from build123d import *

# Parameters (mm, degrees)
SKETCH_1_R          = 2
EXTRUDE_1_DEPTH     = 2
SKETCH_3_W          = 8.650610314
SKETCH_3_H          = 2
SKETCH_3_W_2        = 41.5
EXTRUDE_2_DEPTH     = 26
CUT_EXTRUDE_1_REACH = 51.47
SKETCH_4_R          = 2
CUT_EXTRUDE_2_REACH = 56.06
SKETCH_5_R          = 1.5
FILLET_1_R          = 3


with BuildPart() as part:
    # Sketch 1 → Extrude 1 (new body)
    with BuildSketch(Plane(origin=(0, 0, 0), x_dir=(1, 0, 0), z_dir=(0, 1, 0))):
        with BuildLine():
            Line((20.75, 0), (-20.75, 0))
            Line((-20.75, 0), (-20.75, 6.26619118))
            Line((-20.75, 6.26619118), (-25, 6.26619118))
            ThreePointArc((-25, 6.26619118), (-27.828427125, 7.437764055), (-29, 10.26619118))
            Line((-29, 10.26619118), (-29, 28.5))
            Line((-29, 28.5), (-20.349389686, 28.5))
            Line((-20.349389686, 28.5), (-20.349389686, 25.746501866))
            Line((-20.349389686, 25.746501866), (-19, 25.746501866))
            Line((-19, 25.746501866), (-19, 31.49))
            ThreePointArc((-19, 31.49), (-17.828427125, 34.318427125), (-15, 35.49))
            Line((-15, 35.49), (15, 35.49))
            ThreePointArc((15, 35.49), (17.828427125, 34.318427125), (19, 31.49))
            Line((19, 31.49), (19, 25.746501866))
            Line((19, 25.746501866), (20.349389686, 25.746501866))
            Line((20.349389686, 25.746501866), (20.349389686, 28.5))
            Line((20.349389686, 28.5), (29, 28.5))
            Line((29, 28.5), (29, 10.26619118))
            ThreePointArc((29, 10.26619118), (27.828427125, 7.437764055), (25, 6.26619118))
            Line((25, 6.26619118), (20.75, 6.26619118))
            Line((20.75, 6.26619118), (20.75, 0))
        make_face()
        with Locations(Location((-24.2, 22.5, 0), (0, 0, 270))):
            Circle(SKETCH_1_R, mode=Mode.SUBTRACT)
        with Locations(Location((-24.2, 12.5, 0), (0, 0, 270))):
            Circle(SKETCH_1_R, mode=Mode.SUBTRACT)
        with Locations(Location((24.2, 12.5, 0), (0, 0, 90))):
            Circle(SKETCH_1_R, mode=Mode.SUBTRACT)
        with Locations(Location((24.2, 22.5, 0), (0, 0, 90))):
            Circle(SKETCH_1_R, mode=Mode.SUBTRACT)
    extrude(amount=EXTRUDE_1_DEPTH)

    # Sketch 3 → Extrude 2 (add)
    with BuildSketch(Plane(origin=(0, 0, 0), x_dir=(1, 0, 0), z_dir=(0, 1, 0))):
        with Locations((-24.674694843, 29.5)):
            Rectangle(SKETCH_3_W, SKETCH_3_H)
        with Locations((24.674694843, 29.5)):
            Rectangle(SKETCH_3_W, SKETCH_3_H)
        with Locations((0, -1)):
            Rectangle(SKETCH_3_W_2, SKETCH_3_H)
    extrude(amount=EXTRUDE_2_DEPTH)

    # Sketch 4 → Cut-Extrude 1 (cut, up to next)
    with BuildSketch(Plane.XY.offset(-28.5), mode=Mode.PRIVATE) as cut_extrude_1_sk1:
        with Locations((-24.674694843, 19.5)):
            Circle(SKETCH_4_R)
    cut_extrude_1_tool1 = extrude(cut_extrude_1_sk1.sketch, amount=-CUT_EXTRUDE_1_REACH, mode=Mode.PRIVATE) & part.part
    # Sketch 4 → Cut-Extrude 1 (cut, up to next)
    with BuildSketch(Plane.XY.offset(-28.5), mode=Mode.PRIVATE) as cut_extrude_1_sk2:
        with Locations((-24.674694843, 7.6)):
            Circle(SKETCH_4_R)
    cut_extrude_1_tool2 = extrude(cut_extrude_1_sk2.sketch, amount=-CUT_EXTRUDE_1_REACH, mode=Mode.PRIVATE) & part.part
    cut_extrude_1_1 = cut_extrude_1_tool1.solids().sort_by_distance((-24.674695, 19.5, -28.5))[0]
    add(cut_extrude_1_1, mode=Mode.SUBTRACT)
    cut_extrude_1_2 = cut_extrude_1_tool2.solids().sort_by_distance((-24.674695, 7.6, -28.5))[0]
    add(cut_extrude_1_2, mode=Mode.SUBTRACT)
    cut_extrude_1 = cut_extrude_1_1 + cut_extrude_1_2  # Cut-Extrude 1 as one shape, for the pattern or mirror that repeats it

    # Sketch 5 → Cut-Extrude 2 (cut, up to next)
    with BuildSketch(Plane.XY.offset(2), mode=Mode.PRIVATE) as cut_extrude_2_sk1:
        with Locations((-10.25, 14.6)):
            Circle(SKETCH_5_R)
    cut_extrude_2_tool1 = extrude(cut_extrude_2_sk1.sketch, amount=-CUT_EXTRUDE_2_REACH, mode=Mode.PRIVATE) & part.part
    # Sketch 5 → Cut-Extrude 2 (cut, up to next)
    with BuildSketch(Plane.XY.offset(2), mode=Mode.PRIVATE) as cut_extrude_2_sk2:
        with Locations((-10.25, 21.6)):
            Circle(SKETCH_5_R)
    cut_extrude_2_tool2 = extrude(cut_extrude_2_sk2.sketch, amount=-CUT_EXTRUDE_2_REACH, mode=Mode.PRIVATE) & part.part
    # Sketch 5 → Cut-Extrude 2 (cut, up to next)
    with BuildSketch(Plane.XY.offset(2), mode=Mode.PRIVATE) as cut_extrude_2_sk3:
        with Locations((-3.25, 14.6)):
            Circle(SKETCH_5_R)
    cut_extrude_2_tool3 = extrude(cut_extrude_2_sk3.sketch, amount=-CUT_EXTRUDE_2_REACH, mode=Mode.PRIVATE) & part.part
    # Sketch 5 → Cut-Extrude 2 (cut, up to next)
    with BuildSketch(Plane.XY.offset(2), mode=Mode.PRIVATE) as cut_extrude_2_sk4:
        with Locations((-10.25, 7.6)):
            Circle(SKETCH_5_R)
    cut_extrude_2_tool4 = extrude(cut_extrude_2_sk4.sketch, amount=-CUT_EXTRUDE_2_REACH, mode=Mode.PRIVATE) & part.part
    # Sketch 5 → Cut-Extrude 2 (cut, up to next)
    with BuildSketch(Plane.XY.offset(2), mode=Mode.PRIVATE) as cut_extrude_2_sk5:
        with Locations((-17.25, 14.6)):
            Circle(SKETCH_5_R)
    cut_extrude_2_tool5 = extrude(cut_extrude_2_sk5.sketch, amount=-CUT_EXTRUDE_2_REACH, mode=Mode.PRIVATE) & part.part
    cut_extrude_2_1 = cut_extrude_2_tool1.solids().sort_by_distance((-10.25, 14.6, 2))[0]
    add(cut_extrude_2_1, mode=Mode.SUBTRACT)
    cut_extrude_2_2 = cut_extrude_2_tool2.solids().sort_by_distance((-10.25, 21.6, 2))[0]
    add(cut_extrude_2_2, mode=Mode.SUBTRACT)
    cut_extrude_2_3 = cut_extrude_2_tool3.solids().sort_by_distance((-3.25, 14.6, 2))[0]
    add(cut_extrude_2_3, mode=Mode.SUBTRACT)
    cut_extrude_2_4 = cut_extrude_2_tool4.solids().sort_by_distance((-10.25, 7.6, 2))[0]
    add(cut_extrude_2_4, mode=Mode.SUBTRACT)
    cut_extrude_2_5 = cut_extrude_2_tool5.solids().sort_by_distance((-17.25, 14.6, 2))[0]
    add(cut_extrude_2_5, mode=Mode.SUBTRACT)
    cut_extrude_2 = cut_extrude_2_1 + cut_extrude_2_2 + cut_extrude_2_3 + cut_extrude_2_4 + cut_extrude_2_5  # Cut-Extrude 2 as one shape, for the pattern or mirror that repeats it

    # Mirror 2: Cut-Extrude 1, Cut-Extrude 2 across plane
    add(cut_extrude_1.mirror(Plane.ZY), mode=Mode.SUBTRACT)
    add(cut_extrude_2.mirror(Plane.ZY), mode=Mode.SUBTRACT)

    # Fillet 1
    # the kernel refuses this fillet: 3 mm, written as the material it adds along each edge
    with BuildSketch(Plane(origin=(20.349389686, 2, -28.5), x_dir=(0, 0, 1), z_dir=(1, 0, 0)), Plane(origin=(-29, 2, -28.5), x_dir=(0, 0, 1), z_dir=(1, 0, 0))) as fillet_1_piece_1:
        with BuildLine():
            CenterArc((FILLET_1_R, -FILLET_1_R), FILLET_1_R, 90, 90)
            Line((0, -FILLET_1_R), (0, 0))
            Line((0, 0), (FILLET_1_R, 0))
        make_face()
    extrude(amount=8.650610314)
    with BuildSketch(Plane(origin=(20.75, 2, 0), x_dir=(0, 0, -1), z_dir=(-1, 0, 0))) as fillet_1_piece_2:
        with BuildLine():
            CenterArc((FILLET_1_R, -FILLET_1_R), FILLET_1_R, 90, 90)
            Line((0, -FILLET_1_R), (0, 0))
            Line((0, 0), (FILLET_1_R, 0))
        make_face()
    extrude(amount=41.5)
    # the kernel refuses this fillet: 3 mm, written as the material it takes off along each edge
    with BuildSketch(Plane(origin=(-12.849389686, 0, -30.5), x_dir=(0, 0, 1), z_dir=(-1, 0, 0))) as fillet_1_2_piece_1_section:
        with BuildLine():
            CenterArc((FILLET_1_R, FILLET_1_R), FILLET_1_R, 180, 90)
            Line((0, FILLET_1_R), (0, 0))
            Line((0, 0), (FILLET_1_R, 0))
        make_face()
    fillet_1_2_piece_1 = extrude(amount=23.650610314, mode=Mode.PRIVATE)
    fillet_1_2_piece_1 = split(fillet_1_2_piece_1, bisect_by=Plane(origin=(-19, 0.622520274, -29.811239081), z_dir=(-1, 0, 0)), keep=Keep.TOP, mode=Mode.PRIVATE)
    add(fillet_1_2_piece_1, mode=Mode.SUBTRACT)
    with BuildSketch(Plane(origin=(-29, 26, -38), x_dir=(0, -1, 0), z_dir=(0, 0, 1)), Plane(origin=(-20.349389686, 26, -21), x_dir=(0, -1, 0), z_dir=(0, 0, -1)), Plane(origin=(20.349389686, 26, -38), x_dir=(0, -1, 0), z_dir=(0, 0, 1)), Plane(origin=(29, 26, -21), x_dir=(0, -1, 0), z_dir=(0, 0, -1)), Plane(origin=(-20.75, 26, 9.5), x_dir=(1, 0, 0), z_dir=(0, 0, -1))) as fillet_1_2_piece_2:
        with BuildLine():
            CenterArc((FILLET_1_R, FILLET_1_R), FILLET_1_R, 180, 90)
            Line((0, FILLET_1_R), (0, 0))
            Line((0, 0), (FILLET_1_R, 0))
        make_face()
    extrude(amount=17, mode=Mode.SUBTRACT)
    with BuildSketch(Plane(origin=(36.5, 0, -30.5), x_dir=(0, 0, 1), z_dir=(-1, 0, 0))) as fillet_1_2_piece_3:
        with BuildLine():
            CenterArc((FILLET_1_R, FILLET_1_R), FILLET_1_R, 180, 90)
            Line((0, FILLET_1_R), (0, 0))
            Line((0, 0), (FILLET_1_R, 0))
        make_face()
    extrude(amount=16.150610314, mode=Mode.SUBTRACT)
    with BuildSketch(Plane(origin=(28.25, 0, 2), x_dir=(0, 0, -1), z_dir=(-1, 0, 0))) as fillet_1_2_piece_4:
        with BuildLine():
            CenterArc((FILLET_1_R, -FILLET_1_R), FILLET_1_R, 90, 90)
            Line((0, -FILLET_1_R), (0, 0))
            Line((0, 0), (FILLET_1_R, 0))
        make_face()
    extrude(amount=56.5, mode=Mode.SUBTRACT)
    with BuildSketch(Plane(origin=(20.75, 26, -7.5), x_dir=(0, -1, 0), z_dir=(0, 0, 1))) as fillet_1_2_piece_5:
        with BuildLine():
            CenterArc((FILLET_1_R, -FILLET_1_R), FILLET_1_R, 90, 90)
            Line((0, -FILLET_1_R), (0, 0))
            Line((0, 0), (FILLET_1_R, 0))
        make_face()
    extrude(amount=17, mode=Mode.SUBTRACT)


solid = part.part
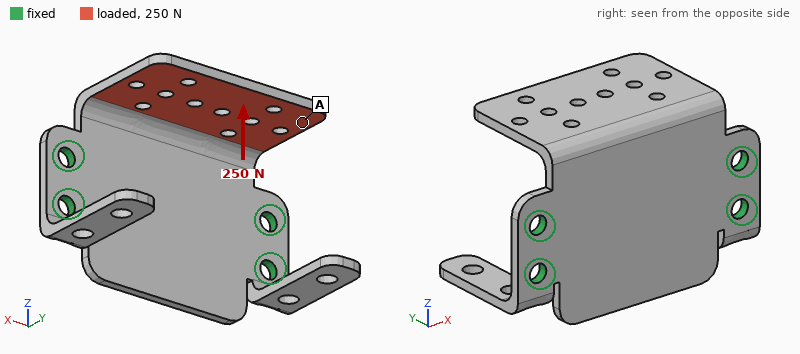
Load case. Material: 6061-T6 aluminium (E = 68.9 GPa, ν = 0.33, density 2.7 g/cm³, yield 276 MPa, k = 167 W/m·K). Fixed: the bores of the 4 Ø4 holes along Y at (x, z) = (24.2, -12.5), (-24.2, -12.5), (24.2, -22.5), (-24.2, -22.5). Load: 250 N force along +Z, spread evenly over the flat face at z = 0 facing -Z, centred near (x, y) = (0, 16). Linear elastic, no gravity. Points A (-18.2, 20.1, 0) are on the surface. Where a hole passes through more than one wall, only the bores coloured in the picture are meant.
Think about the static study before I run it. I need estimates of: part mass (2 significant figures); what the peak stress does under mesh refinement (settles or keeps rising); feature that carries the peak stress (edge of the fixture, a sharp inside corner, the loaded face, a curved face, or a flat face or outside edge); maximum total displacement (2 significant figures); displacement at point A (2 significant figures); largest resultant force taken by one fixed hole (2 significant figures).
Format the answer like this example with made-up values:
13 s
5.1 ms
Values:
17 g
keeps rising
a sharp inside corner
0.86 mm
0.63 mm
120 N
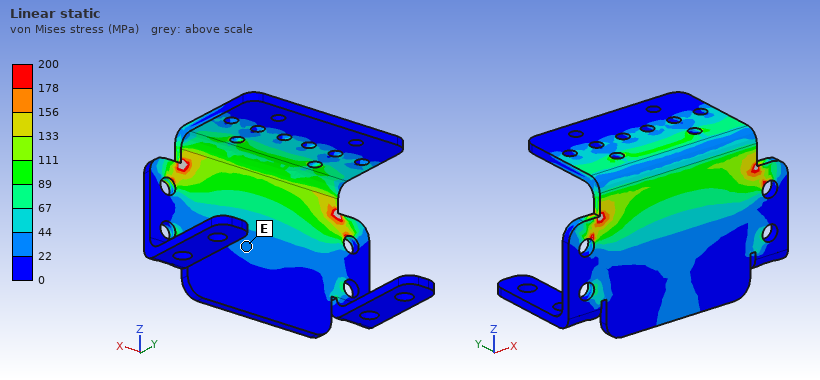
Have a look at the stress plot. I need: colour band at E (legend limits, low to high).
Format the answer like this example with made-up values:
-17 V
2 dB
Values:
22 to 44 MPa
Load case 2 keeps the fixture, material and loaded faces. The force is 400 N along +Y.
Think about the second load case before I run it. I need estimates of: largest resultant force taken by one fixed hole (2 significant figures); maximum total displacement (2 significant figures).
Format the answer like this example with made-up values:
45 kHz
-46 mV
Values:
300 N
0.52 mm
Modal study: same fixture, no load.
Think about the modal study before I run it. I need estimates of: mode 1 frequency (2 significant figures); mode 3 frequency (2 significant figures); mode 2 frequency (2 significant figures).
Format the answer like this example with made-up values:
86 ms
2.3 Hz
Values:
1500 Hz
2300 Hz
2300 Hz
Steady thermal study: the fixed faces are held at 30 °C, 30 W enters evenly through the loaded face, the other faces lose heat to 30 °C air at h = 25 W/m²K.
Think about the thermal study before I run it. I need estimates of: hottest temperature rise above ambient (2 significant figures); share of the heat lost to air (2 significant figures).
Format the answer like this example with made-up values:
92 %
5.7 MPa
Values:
70 K
12 %
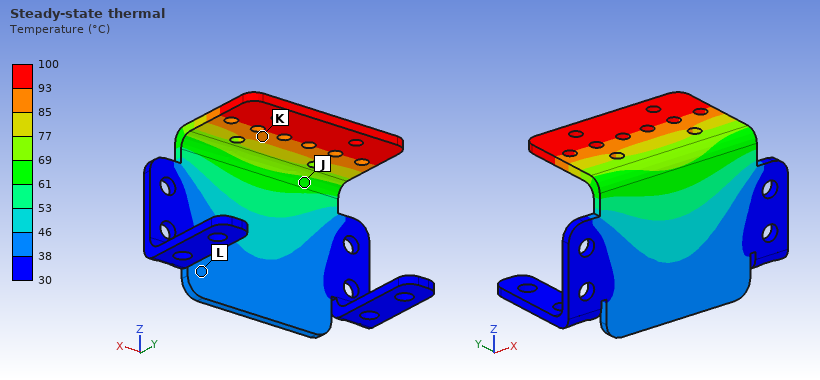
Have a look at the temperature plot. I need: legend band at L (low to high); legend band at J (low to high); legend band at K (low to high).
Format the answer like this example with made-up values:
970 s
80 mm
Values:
38 to 46 °C
61 to 69 °C
85 to 93 °C
